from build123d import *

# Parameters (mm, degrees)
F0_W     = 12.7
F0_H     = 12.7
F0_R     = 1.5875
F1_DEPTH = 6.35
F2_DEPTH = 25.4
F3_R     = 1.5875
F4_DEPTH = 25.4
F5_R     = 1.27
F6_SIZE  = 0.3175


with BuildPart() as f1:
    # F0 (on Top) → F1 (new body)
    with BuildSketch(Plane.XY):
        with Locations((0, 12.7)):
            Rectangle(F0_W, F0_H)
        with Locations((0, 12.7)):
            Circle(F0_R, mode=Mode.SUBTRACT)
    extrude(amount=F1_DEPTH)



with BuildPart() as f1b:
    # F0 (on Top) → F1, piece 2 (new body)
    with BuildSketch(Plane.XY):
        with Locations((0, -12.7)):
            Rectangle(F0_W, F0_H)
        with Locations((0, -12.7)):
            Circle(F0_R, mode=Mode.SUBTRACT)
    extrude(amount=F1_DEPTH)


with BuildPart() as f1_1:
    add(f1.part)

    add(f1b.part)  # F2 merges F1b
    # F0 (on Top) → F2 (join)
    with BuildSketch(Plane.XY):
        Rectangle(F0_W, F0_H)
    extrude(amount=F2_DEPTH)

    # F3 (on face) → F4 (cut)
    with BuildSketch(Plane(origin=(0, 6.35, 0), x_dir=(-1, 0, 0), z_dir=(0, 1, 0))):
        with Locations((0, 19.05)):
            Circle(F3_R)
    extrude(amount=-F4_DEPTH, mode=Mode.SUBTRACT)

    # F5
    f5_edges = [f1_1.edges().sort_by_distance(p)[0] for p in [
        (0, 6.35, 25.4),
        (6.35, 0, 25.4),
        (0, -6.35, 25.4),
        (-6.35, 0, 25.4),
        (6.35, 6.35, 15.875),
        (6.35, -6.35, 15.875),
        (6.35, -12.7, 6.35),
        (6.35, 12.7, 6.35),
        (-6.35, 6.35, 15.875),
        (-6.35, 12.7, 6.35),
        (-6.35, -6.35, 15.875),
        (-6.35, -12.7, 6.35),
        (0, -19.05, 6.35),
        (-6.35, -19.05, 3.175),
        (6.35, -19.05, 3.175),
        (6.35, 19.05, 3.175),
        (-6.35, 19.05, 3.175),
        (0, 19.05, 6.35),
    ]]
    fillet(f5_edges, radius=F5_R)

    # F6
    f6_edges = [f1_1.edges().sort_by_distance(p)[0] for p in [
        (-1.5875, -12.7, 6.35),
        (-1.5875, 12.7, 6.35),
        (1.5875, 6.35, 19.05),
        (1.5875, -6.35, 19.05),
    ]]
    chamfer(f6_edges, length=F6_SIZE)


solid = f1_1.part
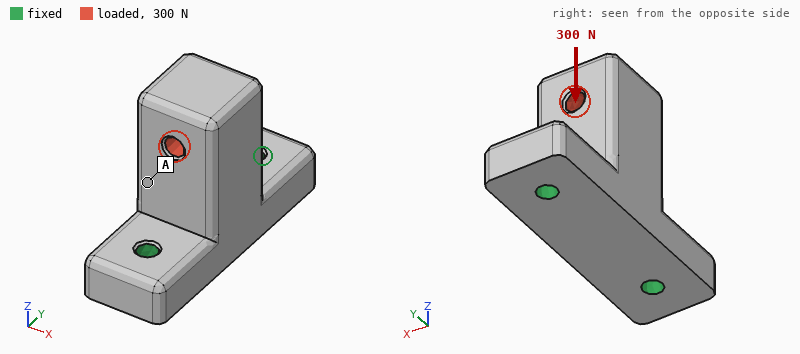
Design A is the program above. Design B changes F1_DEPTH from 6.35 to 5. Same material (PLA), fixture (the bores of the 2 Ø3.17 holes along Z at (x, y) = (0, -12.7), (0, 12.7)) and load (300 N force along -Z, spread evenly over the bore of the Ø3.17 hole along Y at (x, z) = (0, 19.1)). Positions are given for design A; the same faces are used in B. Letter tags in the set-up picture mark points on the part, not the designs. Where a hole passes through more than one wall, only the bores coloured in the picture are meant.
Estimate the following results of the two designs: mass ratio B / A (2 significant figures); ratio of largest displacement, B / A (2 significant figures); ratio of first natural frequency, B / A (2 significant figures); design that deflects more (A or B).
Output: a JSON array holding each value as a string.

["0.93", "1.3", "0.77", "B"]
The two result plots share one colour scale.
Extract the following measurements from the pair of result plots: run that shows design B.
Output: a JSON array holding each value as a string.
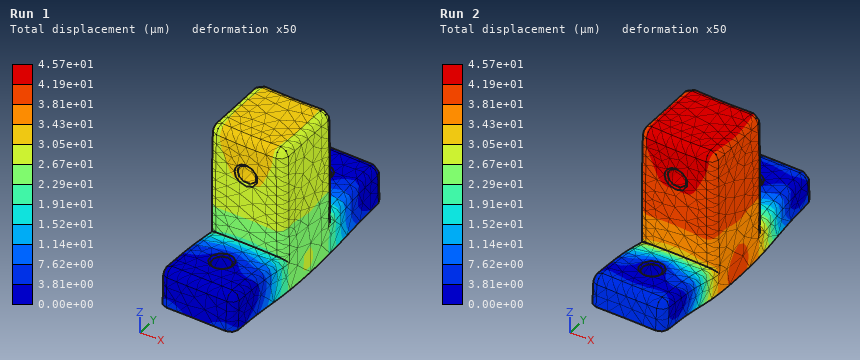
["Run 2"]
